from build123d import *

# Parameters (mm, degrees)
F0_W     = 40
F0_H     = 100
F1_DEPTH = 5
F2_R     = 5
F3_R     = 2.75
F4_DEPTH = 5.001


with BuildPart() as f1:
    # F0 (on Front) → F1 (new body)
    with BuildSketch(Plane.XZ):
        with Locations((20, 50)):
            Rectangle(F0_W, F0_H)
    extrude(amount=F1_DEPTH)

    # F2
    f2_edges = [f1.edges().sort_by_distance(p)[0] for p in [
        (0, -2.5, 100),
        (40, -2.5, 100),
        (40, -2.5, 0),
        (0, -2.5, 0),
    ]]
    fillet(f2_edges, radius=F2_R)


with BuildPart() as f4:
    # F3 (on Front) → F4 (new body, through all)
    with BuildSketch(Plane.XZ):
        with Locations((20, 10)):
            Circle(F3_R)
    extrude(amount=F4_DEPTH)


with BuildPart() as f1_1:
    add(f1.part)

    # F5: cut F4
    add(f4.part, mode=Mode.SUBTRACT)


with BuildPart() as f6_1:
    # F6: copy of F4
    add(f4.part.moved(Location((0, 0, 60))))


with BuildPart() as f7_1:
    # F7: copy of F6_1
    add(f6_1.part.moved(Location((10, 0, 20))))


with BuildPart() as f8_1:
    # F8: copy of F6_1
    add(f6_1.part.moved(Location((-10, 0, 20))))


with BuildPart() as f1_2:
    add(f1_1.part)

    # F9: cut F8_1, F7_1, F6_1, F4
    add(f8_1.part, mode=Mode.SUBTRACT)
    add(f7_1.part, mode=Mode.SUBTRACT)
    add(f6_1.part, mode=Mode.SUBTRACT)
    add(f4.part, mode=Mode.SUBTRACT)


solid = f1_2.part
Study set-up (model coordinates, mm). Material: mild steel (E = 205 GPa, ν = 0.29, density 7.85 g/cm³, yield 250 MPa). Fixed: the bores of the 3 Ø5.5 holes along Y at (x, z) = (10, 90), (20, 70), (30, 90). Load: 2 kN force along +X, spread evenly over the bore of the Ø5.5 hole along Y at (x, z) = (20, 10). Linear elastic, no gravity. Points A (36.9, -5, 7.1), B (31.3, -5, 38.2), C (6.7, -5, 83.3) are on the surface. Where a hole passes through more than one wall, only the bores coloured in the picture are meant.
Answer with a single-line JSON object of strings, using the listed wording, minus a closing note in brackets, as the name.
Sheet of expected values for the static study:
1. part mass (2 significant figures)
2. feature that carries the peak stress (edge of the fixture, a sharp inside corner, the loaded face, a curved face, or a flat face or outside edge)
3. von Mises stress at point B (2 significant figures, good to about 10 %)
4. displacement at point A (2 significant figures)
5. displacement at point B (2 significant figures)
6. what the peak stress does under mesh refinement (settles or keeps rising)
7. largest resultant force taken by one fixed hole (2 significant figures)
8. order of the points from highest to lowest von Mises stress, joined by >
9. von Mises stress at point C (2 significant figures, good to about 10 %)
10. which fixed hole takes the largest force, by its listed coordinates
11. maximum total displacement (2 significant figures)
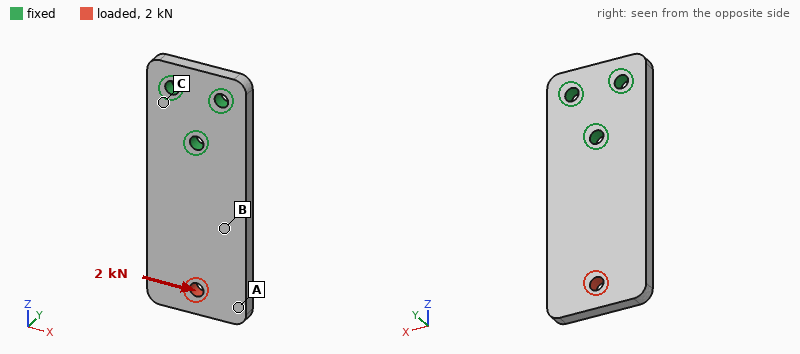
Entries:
{"part mass": "150 g", "feature that carries the peak stress": "edge of the fixture", "von Mises stress at point B": "30 MPa", "displacement at point A": "63 µm", "displacement at point B": "28 µm", "what the peak stress does under mesh refinement": "keeps rising", "largest resultant force taken by one fixed hole": "4.2 kN", "order of the points from highest to lowest von Mises stress, joined by >": "C > B > A", "von Mises stress at point C": "59 MPa", "which fixed hole takes the largest force, by its listed coordinates": "(20, 70)", "maximum total displacement": "70 µm"}
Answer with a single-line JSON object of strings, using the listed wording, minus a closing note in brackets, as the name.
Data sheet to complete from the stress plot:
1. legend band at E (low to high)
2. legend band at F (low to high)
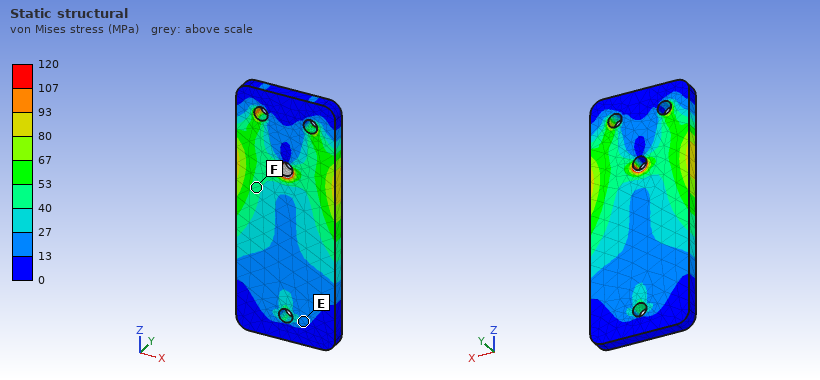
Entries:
{"legend band at E": "13 to 27 MPa", "legend band at F": "40 to 53 MPa"}
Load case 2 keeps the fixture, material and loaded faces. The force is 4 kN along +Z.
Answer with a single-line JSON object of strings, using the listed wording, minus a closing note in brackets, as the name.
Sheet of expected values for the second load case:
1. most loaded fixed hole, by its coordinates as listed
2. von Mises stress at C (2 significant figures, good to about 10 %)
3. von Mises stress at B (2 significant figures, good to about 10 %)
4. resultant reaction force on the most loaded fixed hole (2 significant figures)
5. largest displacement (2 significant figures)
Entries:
{"most loaded fixed hole, by its coordinates as listed": "(20, 70)", "von Mises stress at C": "13 MPa", "von Mises stress at B": "20 MPa", "resultant reaction force on the most loaded fixed hole": "2.5 kN", "largest displacement": "9.4 µm"}
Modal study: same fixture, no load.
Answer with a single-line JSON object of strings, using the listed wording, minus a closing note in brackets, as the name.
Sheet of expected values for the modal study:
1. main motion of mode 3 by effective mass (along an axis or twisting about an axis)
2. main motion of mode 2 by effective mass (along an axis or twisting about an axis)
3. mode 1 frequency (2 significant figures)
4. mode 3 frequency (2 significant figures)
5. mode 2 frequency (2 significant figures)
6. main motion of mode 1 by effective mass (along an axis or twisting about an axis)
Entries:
{"main motion of mode 3 by effective mass": "along X", "main motion of mode 2 by effective mass": "twisting about Z", "mode 1 frequency": "850 Hz", "mode 3 frequency": "4300 Hz", "mode 2 frequency": "2700 Hz", "main motion of mode 1 by effective mass": "along Y"}
